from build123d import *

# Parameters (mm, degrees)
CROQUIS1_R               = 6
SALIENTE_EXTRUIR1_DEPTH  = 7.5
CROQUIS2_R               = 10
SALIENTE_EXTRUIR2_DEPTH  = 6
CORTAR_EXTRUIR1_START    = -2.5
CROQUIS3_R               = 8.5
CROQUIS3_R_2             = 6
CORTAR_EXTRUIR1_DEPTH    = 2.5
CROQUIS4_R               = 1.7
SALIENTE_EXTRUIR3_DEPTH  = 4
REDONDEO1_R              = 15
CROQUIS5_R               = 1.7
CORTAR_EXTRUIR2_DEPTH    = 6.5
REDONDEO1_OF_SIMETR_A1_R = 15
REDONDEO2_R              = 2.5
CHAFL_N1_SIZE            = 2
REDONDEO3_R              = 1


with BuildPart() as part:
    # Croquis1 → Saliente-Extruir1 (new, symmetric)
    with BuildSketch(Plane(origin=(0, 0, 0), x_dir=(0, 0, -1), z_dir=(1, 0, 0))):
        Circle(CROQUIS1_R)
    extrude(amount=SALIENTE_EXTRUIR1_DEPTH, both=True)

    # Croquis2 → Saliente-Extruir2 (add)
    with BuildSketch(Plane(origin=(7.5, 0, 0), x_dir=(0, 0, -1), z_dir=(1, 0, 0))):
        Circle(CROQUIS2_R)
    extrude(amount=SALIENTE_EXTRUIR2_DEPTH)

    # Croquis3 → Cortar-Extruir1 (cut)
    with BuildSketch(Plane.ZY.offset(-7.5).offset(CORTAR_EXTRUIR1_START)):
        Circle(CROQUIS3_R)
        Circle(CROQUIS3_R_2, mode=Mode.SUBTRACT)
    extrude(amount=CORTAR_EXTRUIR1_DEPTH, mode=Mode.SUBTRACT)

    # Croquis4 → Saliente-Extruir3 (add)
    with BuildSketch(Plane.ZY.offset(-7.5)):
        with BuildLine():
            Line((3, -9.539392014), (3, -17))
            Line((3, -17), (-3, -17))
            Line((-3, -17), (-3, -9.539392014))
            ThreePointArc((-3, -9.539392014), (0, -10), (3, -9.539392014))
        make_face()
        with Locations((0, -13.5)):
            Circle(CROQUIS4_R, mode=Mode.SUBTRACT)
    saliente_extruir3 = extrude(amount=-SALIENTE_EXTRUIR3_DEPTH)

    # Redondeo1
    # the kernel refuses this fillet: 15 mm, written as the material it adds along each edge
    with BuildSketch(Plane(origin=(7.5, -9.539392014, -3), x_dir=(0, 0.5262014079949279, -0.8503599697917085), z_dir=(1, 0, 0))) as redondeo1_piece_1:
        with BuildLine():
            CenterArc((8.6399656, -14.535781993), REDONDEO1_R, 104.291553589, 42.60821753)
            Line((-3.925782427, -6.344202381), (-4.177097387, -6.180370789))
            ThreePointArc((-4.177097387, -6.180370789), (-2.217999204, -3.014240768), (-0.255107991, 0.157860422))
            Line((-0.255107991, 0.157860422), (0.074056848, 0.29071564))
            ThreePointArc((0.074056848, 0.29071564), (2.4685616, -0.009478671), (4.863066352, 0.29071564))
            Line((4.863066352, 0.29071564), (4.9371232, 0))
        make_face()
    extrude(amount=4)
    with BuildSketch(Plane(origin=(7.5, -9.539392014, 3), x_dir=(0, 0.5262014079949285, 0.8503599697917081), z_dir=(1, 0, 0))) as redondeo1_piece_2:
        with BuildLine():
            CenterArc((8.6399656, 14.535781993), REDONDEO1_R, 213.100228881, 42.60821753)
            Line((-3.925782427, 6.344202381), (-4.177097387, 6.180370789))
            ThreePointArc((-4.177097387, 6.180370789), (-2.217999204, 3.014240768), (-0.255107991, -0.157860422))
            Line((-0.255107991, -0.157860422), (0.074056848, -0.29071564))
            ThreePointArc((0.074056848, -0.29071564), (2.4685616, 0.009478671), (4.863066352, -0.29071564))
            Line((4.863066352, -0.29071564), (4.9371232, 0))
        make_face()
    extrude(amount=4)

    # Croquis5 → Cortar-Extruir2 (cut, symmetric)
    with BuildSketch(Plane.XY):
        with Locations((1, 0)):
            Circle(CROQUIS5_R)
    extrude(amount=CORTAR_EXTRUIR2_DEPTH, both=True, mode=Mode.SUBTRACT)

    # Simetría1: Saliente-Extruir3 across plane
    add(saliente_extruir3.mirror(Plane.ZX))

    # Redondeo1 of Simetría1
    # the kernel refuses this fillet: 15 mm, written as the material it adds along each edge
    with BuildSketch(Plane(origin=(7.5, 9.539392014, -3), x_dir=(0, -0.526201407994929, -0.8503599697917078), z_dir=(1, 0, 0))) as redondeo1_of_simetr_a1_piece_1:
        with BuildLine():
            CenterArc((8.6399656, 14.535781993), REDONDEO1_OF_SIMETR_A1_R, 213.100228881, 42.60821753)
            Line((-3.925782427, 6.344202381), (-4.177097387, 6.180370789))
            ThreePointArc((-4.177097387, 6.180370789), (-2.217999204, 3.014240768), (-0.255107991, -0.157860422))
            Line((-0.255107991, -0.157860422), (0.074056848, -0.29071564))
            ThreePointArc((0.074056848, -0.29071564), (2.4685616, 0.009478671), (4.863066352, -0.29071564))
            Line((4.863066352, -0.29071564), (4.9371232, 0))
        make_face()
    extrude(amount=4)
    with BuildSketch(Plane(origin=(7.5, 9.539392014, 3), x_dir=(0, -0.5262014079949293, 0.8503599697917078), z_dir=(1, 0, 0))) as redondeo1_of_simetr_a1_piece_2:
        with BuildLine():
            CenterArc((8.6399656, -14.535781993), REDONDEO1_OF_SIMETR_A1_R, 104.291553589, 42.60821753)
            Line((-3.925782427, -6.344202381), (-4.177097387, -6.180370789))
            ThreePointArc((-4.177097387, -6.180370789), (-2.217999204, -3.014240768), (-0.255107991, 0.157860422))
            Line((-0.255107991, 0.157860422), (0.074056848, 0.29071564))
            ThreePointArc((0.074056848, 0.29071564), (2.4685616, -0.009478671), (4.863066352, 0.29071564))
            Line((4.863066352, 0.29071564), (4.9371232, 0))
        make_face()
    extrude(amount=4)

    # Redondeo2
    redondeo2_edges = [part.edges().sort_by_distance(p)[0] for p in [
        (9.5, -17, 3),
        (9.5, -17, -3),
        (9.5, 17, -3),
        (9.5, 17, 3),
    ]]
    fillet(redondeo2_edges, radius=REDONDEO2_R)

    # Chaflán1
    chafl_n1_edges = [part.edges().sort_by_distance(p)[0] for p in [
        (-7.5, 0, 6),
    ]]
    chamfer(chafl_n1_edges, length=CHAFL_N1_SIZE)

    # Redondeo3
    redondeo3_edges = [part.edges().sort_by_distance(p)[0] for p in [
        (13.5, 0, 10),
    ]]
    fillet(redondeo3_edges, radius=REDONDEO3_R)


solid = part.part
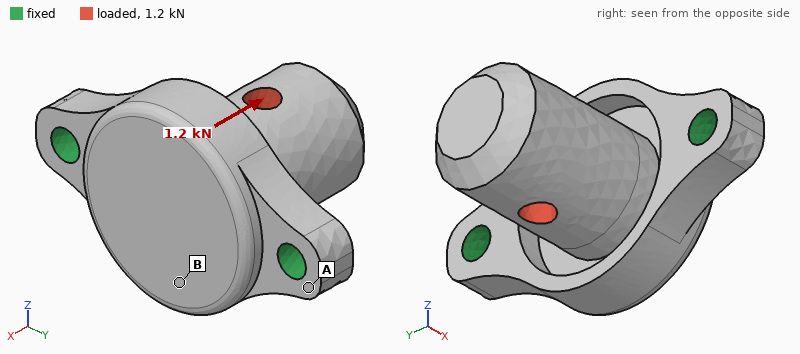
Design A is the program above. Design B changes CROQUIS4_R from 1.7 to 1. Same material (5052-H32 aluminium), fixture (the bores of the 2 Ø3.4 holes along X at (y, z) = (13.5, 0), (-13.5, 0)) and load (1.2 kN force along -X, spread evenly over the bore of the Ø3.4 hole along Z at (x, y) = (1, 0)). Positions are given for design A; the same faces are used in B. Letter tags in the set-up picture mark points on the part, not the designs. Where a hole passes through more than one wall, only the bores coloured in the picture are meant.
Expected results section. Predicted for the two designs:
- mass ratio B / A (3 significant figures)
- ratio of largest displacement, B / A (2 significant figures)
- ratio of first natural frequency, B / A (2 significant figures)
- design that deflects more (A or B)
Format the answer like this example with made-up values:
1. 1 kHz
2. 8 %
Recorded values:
1. 1.01
2. 1.3
3. 0.90
4. B
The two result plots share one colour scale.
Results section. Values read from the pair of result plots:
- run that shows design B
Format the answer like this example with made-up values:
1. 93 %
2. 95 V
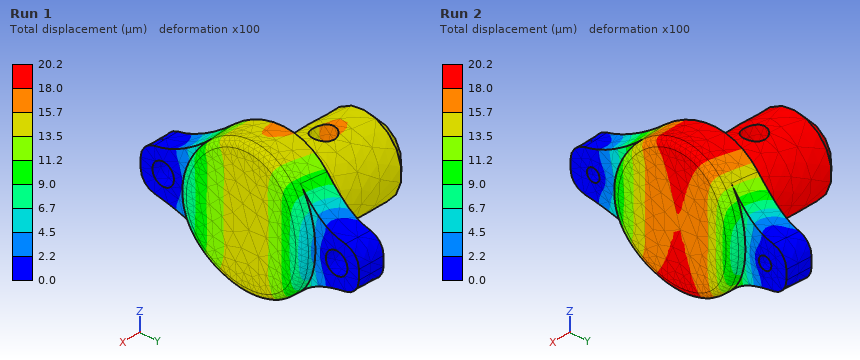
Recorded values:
1. Run 2
